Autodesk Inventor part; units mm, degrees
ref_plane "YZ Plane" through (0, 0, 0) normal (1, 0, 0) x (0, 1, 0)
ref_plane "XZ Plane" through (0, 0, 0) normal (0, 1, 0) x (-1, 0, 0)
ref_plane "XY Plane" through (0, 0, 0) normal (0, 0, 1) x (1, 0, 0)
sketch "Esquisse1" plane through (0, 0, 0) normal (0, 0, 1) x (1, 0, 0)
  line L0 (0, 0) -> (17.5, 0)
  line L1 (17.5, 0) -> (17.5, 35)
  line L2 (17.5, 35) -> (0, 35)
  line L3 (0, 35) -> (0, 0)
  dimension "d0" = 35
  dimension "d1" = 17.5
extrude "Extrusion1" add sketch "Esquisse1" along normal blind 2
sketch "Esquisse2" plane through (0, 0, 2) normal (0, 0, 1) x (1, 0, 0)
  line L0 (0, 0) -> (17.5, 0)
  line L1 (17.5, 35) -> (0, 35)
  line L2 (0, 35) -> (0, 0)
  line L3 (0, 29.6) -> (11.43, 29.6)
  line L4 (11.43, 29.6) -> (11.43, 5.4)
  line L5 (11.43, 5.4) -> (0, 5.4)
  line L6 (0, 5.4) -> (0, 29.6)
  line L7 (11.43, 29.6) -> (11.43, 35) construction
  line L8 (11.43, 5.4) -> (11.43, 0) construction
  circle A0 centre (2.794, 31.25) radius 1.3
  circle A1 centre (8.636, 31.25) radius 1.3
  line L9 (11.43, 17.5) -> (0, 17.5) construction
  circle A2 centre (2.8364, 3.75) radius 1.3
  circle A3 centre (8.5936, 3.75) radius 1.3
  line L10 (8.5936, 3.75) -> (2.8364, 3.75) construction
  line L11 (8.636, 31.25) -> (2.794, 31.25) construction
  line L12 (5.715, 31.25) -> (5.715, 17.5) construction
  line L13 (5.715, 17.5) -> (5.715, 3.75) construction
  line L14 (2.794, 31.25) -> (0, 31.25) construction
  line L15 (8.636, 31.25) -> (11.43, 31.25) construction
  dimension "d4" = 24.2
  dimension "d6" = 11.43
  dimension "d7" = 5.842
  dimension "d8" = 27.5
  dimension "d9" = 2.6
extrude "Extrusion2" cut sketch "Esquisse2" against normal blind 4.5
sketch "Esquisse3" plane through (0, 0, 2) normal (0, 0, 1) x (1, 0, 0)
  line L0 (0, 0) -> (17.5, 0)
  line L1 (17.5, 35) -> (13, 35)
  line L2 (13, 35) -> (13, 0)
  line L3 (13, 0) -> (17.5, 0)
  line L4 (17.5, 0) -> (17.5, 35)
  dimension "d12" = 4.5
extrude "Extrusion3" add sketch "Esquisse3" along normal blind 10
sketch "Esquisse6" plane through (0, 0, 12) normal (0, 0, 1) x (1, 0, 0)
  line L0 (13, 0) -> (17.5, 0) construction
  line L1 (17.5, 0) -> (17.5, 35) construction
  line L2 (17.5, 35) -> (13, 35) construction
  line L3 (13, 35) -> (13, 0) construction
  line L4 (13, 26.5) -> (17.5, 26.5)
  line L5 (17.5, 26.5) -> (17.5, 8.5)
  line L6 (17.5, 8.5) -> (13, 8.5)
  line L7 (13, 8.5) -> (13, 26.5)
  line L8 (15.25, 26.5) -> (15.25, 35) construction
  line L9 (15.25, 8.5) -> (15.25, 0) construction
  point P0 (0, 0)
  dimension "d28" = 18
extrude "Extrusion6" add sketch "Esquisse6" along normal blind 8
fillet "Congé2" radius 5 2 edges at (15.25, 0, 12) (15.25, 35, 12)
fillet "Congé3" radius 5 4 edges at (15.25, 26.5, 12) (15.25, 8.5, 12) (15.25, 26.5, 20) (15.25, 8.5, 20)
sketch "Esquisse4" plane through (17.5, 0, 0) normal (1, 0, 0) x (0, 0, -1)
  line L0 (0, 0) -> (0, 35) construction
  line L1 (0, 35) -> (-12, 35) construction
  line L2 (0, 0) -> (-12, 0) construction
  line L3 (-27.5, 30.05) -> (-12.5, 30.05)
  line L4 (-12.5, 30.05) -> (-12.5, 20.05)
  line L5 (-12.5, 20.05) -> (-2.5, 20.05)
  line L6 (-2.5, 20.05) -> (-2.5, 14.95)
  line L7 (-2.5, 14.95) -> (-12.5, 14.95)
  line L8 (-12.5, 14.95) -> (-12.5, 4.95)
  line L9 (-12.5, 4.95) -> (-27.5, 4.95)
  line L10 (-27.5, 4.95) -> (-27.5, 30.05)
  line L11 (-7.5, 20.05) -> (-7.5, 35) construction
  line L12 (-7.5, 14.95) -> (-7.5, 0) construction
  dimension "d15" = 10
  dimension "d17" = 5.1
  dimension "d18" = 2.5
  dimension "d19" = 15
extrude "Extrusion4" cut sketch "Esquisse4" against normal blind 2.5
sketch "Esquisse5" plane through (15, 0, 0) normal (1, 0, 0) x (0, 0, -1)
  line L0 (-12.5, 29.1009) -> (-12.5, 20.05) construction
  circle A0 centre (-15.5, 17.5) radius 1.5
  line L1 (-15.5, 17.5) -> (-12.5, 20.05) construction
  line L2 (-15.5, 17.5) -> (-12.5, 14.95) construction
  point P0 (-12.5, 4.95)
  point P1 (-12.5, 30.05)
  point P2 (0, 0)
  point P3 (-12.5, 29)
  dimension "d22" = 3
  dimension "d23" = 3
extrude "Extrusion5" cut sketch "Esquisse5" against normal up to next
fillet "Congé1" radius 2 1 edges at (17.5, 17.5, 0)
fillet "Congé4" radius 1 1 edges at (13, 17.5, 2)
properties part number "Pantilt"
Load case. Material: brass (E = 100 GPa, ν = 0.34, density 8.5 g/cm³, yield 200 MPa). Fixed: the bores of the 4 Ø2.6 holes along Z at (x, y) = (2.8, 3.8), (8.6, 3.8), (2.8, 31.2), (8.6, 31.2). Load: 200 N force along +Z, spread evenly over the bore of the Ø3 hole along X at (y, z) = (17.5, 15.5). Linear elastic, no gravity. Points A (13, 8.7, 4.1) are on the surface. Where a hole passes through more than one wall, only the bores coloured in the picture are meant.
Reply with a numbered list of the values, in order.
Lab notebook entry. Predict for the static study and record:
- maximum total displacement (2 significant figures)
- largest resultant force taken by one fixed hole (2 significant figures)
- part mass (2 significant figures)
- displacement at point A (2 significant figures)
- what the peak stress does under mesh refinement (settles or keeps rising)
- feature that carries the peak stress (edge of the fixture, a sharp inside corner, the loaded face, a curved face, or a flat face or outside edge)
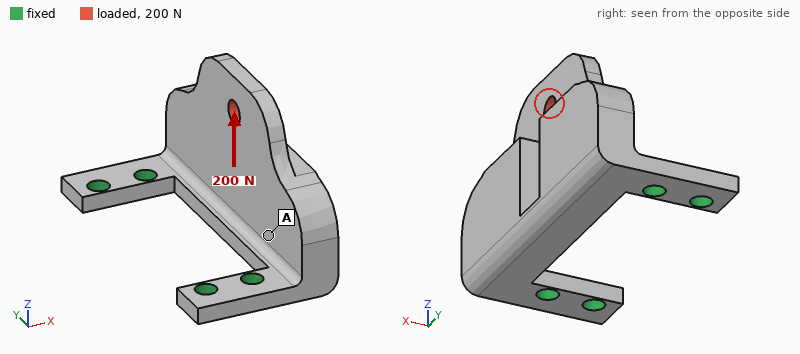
1. 51 µm
2. 110 N
3. 20 g
4. 11 µm
5. keeps rising
6. edge of the fixture
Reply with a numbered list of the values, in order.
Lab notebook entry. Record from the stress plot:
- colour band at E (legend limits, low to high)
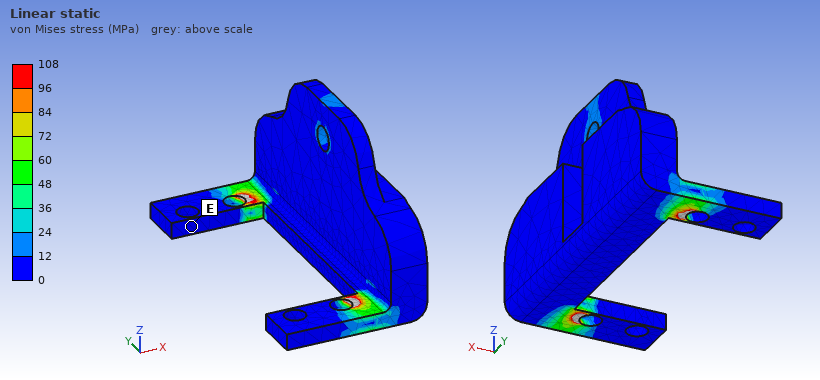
1. 0 to 12 MPa
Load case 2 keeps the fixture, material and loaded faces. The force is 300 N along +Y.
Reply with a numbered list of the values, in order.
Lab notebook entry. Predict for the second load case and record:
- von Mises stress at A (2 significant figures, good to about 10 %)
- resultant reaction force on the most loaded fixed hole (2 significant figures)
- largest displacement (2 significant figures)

1. 20 MPa
2. 230 N
3. 15 µm
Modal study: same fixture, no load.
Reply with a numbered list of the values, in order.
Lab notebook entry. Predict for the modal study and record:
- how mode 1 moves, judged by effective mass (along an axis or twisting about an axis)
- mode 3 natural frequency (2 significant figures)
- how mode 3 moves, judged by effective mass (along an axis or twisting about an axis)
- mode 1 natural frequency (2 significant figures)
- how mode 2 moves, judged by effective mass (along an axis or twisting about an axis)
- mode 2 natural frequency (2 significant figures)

1. along X
2. 8900 Hz
3. along Z
4. 1900 Hz
5. along Y
6. 7300 Hz
